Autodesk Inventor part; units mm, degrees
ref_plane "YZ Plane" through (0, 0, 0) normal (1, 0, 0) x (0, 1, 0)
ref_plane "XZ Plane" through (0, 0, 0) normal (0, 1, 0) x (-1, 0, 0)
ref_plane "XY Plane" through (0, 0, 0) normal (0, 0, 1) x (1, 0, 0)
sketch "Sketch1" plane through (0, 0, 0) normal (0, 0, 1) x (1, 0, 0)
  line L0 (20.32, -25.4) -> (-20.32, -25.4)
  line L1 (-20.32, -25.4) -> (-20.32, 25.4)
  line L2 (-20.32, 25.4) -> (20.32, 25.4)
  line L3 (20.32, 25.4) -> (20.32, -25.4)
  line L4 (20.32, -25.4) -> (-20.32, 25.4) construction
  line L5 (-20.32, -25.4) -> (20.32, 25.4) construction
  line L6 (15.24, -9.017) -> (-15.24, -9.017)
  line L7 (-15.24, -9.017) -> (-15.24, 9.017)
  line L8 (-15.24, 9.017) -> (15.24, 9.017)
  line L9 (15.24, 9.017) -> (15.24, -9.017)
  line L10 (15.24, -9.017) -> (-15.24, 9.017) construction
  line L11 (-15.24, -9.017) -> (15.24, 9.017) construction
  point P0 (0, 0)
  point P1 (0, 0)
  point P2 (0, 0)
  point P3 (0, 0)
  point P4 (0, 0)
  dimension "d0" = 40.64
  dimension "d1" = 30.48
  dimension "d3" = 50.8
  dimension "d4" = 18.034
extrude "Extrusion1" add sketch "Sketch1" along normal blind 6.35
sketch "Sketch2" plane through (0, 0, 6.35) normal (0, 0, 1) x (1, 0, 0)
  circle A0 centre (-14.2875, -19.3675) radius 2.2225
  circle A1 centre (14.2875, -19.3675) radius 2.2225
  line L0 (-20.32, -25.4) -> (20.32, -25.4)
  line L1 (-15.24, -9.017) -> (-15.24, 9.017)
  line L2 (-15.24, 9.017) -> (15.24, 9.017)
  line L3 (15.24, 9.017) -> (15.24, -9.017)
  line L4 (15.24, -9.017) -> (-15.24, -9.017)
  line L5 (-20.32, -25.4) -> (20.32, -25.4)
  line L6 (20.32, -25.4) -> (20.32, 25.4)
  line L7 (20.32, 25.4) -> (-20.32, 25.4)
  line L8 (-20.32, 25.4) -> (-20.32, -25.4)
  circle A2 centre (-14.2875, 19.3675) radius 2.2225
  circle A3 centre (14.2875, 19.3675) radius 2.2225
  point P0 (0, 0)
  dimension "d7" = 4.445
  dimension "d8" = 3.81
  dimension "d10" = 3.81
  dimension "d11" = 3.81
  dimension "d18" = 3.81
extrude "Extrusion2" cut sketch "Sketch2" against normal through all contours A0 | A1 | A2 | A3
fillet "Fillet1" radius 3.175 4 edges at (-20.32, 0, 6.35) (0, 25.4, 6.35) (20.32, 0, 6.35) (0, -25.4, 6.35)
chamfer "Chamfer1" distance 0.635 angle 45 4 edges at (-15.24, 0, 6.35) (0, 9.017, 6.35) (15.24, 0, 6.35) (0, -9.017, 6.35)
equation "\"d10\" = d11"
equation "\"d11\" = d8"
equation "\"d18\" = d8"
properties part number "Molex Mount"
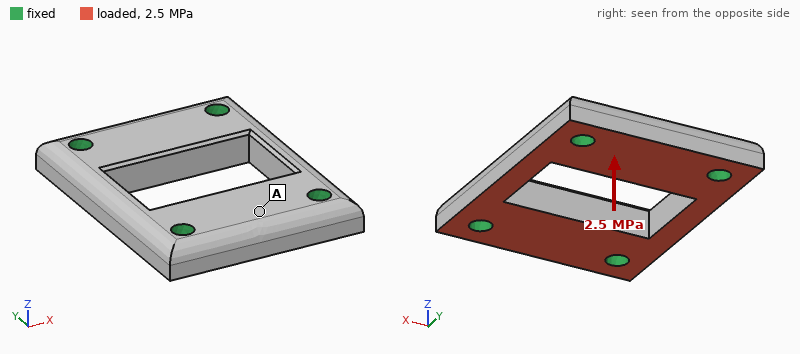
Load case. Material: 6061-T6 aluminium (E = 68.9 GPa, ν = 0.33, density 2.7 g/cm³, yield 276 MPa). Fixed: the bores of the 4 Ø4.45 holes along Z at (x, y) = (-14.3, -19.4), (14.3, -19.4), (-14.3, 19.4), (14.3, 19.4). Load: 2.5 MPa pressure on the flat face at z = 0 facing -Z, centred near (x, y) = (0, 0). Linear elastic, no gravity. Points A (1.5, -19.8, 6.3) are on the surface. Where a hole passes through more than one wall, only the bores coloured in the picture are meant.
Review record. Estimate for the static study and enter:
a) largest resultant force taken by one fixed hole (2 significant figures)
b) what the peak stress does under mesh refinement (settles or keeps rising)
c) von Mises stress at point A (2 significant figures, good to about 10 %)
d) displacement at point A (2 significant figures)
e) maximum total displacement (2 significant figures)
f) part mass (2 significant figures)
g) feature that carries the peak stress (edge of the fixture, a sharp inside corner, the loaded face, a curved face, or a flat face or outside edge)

910 N
keeps rising
11 MPa
4.1 µm
9.9 µm
24 g
edge of the fixture
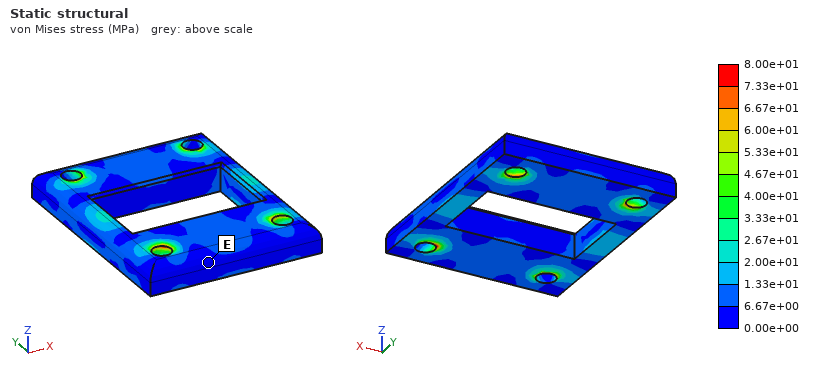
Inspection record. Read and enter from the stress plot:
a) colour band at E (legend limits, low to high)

0.00e+00 to 6.67e+00 MPa
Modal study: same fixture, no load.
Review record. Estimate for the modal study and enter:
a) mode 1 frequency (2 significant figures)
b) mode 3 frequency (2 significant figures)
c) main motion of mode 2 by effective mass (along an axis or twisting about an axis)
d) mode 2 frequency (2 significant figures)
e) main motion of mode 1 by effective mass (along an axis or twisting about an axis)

24 kHz
28 kHz
twisting about Y
25 kHz
along Z
